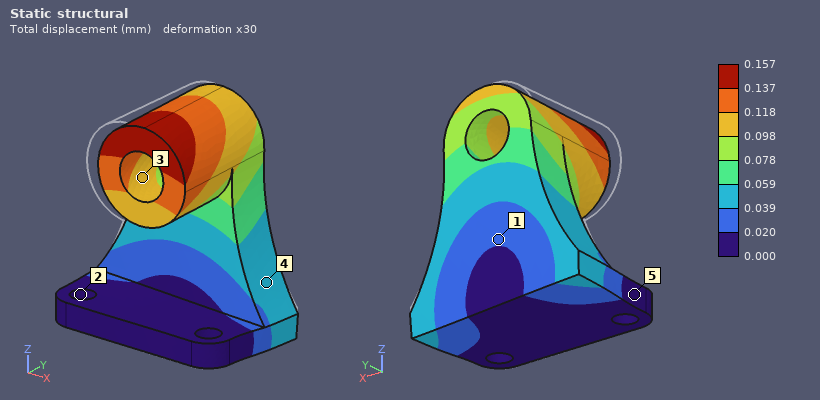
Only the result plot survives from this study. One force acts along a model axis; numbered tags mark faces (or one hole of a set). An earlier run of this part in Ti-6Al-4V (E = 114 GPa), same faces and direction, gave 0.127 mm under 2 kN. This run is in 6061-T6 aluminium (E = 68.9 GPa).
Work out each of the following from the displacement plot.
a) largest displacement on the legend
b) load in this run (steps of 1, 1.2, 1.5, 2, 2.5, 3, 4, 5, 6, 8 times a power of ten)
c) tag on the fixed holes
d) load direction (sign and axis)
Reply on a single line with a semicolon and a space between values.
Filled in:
0.157 mm; 1.5 kN; 2; +X
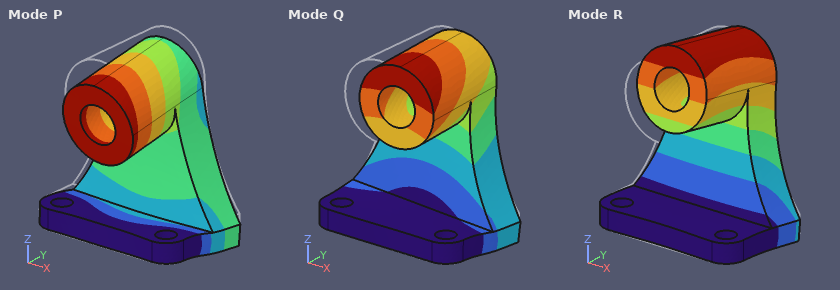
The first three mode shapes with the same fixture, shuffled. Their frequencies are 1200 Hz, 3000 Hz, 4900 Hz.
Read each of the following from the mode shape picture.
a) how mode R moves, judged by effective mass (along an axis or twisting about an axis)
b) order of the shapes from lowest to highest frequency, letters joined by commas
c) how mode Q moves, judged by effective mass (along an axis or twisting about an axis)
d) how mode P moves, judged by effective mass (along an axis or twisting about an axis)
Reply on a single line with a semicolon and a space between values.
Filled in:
along Y; R, Q, P; along X; along Z
